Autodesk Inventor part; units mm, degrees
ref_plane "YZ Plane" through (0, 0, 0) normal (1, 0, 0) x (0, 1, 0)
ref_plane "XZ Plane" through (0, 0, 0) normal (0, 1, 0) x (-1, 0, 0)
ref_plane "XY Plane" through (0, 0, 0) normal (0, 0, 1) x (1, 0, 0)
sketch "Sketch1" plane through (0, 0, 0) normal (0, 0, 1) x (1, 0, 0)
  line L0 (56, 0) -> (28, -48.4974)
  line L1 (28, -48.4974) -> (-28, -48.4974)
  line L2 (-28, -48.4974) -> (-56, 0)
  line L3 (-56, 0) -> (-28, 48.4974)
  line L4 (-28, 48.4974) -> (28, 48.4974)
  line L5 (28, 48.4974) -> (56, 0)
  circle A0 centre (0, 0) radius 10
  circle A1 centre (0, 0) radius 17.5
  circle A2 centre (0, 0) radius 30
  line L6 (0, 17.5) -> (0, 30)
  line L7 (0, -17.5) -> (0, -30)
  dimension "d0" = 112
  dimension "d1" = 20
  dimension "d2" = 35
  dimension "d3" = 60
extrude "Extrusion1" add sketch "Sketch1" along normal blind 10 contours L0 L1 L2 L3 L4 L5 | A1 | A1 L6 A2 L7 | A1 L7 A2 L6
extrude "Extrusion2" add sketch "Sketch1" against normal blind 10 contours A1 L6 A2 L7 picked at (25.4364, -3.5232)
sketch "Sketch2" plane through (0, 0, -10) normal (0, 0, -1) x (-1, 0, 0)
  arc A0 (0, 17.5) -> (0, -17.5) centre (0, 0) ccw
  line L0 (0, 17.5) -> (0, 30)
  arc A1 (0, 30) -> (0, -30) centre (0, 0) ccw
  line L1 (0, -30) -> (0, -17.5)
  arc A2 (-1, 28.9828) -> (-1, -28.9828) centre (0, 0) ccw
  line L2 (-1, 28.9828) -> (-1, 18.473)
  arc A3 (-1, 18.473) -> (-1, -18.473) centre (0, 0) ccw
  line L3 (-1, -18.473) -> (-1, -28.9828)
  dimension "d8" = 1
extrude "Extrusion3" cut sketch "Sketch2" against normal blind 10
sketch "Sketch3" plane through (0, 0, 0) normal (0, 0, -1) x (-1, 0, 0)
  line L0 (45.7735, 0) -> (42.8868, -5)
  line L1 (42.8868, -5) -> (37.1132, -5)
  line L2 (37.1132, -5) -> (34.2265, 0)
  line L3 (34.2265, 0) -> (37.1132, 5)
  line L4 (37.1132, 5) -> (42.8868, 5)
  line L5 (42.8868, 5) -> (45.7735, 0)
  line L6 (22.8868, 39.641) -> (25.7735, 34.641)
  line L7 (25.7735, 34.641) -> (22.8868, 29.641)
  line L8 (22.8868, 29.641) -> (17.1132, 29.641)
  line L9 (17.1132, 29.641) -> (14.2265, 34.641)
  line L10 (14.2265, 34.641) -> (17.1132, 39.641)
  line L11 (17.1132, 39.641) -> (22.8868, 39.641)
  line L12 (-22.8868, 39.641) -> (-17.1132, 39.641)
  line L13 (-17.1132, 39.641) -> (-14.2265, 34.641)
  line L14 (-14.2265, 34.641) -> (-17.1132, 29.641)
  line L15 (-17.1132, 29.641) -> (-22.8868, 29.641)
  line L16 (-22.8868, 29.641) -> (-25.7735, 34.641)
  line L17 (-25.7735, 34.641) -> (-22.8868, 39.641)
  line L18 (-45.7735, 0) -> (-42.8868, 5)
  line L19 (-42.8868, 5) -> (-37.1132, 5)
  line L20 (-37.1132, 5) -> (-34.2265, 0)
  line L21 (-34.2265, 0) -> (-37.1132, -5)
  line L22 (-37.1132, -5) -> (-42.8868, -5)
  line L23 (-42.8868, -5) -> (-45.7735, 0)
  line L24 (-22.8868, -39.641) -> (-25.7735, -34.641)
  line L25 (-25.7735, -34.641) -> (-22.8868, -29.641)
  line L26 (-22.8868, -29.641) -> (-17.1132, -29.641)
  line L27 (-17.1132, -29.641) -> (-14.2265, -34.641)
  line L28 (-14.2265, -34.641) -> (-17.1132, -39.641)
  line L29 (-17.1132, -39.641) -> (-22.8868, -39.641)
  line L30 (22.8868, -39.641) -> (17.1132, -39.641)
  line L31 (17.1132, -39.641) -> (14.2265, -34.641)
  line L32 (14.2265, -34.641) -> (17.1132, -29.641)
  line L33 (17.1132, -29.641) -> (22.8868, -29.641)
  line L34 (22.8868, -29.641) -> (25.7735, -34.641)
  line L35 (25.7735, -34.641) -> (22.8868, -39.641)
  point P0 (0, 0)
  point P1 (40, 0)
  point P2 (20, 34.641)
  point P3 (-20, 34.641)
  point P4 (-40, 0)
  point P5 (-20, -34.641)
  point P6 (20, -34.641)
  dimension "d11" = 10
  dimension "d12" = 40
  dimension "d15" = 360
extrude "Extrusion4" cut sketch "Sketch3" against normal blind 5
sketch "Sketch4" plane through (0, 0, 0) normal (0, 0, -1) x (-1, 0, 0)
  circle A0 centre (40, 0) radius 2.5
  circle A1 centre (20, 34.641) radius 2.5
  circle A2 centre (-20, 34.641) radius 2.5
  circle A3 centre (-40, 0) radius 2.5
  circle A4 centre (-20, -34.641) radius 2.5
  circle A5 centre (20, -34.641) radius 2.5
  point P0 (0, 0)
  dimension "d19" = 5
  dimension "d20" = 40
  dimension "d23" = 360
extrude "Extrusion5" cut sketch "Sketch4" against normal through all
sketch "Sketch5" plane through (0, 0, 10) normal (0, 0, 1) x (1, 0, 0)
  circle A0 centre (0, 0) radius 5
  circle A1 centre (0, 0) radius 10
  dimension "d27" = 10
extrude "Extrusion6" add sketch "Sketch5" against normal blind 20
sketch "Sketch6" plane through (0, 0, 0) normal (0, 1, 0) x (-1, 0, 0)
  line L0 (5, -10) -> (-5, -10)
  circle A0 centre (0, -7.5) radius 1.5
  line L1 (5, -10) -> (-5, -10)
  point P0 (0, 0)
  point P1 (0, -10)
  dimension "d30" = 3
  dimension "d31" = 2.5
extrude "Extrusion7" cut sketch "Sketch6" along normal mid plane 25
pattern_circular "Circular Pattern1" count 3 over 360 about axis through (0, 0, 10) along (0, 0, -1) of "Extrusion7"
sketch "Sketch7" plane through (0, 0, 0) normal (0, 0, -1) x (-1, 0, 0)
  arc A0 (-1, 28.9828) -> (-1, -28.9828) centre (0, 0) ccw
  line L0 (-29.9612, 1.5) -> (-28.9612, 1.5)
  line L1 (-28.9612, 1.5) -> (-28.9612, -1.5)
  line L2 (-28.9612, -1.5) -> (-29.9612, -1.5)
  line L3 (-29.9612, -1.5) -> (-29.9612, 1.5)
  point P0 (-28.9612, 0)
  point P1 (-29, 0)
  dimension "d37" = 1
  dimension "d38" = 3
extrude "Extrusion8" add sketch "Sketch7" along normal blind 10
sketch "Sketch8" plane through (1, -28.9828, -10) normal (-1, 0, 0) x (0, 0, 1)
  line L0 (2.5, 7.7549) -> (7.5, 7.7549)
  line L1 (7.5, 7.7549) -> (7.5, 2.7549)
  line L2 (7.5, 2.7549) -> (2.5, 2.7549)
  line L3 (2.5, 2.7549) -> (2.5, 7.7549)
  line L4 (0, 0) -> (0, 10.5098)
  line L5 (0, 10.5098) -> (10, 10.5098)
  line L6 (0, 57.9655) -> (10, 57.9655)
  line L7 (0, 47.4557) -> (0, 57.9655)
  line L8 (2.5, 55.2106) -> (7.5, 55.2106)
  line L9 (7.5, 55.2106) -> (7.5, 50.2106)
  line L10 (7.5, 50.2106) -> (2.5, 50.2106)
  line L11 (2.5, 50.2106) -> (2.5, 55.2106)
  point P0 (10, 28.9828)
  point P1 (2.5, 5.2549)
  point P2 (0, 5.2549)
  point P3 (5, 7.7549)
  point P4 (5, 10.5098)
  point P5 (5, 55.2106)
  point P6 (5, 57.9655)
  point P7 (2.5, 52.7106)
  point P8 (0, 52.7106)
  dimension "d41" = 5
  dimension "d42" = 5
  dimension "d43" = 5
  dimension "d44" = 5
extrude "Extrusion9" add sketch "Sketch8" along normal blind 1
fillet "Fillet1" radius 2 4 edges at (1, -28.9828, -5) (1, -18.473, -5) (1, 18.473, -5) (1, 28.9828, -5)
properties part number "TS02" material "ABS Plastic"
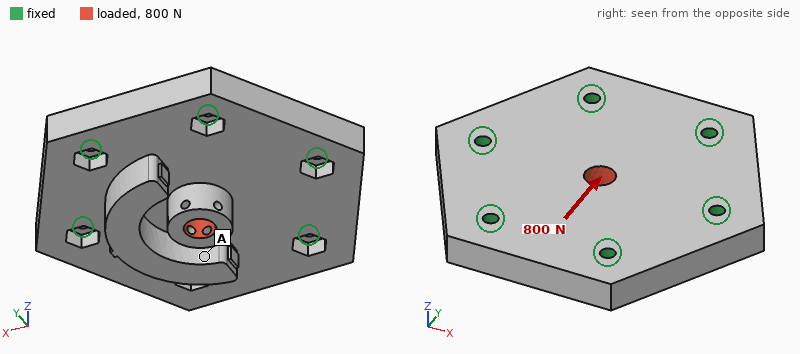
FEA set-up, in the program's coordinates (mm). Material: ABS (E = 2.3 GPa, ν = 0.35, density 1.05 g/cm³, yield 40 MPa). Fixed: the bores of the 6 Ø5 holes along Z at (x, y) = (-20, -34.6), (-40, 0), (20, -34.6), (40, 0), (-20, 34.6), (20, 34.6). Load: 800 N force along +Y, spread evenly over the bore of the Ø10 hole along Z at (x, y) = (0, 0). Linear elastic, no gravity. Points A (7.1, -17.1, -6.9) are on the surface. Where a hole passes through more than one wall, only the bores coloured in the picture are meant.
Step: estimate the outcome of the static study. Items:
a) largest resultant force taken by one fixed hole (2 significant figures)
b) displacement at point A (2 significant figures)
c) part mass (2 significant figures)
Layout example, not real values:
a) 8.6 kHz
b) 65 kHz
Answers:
a) 180 N
b) 12 µm
c) 92 g
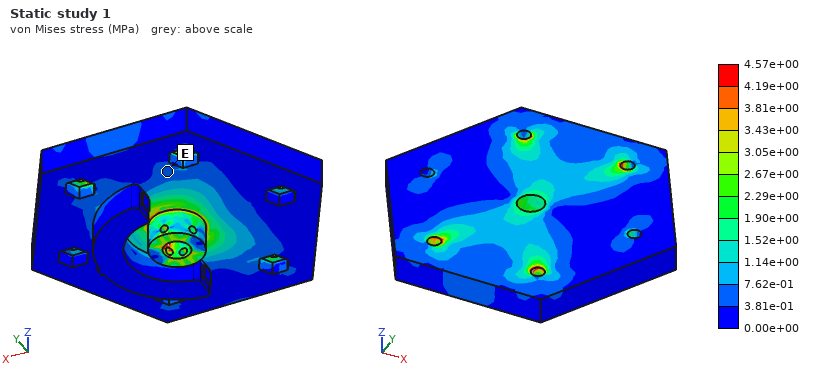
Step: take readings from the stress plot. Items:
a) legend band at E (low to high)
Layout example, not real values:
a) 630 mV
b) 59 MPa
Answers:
a) 3.81e-01 to 7.62e-01 MPa
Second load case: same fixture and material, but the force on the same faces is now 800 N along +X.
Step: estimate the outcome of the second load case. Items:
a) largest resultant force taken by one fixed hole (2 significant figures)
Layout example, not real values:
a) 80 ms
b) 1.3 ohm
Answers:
a) 210 N
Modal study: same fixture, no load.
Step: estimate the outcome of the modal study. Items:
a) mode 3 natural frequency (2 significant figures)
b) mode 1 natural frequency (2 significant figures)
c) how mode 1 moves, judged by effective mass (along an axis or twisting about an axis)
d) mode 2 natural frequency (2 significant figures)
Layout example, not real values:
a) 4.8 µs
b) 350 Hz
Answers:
a) 4600 Hz
b) 2700 Hz
c) along Z
d) 4500 Hz
